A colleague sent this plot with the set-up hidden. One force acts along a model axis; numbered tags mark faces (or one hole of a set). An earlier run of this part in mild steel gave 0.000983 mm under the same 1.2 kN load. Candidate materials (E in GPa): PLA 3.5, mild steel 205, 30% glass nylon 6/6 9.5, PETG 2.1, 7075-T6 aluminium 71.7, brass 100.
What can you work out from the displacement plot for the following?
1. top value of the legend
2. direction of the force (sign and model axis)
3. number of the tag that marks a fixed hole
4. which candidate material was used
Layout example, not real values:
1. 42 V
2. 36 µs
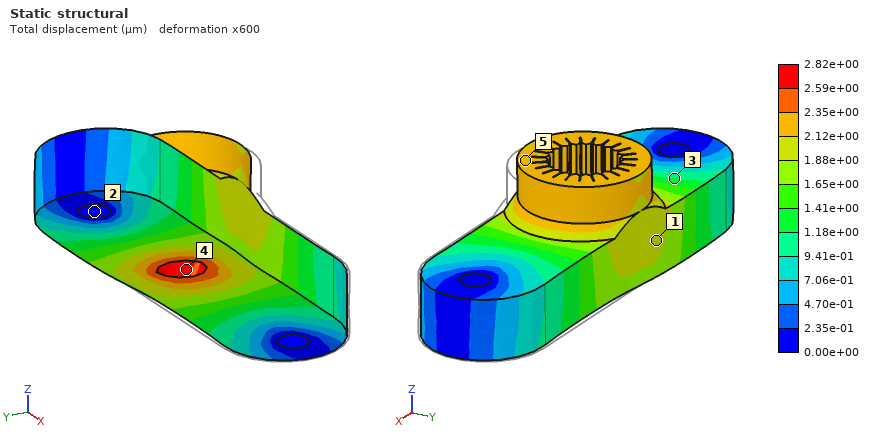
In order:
1. 2.82e+00 µm
2. -X
3. 2
4. 7075-T6 aluminium
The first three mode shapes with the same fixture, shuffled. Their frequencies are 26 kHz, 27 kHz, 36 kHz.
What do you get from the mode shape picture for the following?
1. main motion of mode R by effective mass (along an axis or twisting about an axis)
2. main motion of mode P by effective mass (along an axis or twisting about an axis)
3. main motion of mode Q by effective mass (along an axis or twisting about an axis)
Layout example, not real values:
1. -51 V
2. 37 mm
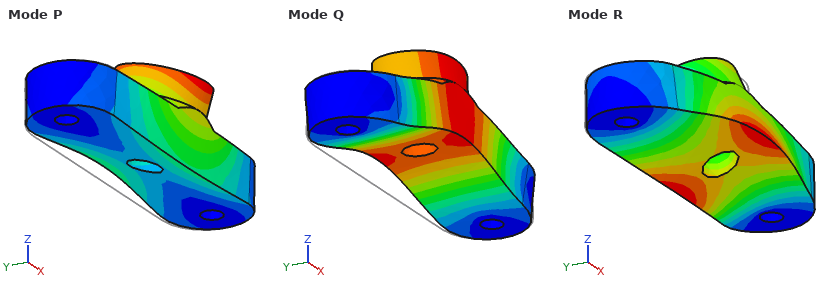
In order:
1. along Y
2. along Y
3. along Z
